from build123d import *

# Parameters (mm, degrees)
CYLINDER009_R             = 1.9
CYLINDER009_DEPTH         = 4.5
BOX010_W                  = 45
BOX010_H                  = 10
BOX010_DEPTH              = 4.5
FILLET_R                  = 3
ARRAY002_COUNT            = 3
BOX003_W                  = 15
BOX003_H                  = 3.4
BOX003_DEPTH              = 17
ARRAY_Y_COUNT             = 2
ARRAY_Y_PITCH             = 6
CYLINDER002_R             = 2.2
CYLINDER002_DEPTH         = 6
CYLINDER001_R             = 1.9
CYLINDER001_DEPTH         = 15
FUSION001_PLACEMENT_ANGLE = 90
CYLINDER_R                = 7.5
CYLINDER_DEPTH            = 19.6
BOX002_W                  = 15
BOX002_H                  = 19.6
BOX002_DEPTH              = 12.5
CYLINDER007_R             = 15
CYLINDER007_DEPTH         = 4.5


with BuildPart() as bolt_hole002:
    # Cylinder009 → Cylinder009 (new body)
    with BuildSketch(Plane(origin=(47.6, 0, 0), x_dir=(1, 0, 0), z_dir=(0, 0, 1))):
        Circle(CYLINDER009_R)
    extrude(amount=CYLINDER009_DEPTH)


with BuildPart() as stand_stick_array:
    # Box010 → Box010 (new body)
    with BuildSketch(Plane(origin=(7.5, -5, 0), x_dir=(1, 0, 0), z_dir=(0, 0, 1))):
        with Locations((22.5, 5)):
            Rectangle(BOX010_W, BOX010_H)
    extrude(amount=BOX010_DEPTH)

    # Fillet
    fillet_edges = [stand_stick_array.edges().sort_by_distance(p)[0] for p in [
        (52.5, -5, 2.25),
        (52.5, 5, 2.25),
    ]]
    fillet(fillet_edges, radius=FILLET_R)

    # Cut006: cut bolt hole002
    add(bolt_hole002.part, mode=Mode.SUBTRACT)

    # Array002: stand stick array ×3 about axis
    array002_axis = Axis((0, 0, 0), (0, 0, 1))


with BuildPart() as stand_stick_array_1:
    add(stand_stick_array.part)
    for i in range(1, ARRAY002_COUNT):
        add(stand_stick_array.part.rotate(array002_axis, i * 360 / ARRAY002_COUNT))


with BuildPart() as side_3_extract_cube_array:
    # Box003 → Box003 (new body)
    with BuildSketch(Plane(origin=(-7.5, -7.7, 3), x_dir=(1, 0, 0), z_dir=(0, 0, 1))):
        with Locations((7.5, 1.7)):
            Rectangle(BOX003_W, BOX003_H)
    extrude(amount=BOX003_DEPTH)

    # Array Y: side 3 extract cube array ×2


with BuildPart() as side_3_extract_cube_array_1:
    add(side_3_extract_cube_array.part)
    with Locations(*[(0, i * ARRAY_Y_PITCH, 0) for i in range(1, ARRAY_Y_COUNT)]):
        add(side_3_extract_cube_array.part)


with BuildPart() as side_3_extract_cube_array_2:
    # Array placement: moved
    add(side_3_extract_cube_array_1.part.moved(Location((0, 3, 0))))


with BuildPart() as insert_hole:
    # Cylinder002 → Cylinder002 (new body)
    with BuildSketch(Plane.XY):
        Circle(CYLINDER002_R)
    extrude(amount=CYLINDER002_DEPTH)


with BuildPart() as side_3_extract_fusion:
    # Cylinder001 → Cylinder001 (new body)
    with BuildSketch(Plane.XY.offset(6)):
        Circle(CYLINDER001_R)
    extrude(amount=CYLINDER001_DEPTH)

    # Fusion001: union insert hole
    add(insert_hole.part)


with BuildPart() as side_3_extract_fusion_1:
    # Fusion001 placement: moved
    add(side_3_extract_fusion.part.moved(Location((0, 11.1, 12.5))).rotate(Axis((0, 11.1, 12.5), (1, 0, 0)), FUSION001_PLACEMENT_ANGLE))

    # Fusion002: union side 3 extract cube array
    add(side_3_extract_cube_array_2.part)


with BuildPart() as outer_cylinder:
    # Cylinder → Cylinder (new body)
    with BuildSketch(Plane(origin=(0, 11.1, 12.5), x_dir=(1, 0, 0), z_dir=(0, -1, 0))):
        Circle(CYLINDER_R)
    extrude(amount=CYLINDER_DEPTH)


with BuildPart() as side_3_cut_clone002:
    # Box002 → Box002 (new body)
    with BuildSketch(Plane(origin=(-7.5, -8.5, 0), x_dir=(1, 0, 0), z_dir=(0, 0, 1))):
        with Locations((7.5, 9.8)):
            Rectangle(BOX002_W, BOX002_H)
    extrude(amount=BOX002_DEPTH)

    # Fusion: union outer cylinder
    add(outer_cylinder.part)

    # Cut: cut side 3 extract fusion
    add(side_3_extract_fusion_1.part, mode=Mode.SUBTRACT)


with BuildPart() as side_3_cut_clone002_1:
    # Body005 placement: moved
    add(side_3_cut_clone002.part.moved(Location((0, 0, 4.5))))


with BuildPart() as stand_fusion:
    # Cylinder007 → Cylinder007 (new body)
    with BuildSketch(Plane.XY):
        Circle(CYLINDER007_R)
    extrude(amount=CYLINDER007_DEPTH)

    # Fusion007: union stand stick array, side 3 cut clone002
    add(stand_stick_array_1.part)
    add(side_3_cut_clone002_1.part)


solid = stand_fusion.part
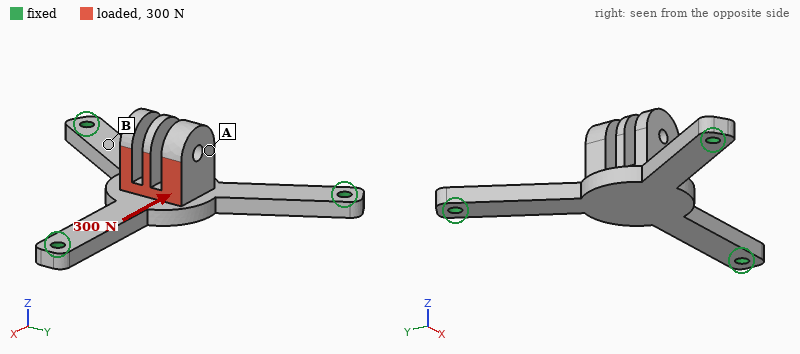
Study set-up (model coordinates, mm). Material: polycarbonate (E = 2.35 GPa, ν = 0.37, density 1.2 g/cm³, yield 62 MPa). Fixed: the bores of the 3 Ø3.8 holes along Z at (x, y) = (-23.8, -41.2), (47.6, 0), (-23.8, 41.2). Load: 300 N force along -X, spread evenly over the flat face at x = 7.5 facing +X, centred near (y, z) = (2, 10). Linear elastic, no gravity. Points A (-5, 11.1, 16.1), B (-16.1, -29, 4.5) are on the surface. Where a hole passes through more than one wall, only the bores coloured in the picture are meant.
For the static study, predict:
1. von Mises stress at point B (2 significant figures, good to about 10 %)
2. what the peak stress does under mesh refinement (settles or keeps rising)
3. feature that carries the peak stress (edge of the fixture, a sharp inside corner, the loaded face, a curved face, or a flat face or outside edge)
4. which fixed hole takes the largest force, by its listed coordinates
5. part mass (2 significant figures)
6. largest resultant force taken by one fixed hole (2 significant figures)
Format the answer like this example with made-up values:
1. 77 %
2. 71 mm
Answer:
1. 6.6 MPa
2. keeps rising
3. edge of the fixture
4. (47.6, 0)
5. 14 g
6. 190 N
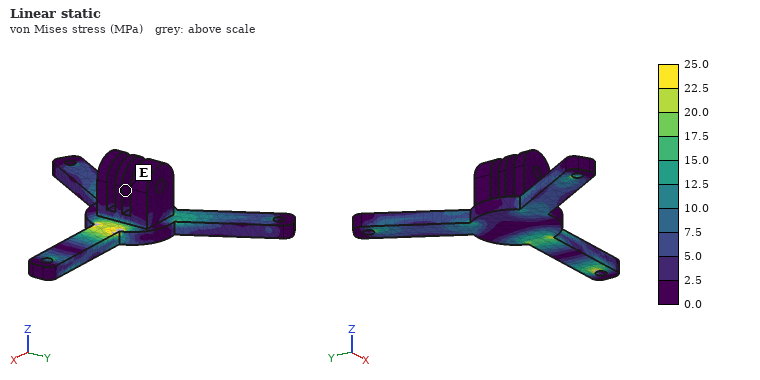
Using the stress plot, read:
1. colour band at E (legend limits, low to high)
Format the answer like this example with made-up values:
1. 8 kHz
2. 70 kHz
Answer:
1. 0.0 to 2.5 MPa
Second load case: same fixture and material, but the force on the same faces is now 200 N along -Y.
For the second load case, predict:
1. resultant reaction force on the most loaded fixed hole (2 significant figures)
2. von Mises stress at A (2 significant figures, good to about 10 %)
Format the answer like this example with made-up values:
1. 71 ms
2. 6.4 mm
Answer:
1. 110 N
2. 1.4 MPa
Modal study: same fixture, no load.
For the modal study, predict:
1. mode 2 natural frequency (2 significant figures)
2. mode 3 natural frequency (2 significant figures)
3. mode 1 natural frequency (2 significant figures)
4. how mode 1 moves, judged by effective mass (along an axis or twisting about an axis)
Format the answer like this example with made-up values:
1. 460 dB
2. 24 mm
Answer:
1. 1100 Hz
2. 1100 Hz
3. 550 Hz
4. along Z
